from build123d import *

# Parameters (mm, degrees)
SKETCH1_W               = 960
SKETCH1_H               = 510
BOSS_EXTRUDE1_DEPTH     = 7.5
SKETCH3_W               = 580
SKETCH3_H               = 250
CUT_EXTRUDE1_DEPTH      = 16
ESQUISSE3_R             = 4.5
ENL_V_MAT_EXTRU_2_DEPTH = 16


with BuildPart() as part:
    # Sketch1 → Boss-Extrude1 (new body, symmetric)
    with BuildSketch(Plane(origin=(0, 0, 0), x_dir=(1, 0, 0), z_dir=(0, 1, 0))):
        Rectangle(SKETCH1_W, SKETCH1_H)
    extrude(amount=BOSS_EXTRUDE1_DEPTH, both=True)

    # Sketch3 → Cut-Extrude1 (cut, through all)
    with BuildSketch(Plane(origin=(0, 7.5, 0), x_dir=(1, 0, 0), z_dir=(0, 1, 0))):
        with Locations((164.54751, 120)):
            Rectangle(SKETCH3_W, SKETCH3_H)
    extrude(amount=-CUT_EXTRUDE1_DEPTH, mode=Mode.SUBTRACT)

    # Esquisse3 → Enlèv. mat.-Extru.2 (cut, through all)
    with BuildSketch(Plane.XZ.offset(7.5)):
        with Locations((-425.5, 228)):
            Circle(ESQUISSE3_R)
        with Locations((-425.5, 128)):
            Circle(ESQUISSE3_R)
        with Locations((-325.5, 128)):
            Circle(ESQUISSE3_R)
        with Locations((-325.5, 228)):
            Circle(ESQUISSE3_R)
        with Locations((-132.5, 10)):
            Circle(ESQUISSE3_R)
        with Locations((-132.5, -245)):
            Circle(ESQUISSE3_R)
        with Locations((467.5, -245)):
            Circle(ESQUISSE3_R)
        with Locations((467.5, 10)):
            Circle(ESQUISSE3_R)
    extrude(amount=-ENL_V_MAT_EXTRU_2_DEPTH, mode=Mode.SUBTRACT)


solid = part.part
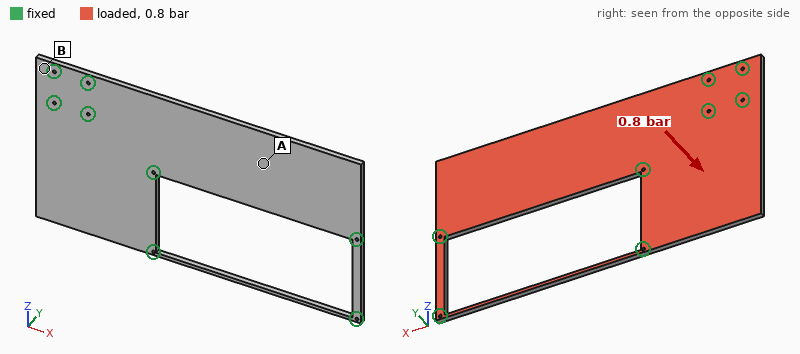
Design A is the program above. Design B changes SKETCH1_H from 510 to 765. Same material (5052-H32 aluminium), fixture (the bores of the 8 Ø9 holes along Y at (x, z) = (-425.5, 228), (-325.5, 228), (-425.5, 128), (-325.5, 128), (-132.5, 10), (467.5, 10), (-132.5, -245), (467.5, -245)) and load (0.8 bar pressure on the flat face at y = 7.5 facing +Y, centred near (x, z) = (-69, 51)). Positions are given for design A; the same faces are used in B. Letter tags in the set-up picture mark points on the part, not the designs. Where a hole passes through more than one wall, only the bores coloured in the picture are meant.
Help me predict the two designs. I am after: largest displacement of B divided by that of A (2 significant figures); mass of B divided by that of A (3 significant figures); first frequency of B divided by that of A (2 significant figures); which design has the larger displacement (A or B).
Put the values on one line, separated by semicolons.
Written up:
2.6; 1.71; 0.64; B
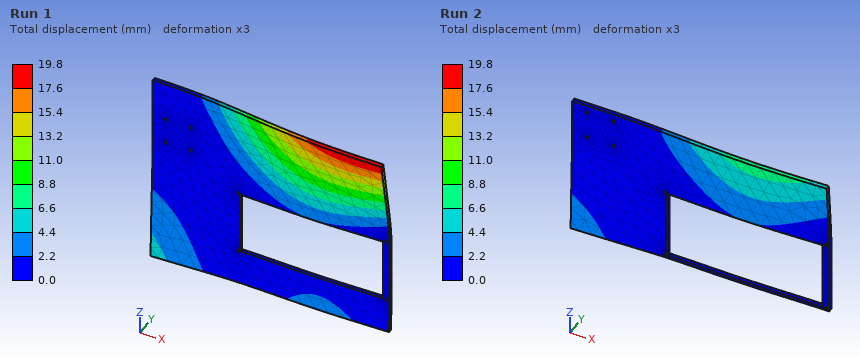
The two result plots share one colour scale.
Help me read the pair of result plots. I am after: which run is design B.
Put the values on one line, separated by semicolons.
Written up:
Run 1
